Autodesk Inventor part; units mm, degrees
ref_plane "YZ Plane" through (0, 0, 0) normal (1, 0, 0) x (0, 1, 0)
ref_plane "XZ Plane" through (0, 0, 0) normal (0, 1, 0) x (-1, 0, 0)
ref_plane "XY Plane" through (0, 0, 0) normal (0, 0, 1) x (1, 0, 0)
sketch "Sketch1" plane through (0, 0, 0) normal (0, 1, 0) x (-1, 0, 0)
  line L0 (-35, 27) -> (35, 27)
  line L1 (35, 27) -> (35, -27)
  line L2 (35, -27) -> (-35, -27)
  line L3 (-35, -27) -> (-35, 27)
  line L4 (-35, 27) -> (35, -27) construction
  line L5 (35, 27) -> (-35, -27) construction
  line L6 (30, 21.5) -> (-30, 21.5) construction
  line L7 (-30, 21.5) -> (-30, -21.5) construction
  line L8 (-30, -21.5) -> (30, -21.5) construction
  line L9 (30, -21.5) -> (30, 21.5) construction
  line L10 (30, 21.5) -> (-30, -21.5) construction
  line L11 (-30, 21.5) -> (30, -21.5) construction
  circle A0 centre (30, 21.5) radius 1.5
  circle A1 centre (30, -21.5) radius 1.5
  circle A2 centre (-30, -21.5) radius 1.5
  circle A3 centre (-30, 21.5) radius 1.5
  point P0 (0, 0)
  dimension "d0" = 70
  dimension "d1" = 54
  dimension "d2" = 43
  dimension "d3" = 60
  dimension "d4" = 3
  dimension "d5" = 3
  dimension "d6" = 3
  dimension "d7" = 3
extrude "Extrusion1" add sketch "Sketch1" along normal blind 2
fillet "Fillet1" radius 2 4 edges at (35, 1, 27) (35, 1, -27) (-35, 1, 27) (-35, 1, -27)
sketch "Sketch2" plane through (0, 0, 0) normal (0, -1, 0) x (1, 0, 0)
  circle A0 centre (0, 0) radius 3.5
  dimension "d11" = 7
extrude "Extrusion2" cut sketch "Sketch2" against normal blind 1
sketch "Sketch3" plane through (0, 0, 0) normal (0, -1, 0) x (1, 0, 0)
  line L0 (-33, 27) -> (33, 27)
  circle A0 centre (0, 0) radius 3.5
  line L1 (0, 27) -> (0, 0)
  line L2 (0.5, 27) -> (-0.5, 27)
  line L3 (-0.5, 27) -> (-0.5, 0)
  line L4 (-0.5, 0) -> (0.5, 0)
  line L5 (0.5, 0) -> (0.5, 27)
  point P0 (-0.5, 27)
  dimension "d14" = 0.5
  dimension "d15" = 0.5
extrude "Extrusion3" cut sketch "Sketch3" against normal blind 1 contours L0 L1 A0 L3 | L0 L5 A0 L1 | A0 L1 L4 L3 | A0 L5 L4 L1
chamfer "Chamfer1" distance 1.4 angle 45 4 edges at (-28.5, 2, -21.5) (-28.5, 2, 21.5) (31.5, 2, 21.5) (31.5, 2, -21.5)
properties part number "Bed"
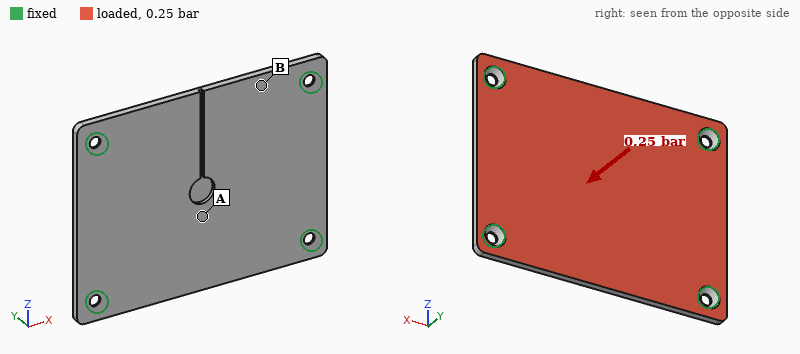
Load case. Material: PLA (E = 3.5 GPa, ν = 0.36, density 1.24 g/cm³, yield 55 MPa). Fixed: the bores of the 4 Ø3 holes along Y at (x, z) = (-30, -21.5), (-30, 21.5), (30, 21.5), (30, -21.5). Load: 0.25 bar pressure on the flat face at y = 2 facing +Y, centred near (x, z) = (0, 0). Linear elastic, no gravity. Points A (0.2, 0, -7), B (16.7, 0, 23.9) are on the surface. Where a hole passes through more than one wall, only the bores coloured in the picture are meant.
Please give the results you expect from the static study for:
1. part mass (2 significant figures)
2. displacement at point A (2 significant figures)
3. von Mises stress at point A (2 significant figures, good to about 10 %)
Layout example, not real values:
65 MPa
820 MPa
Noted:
9.2 g
0.78 mm
8.5 MPa
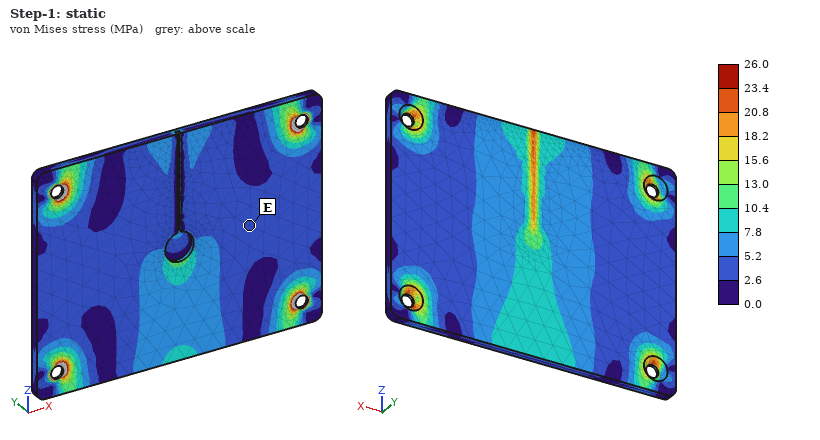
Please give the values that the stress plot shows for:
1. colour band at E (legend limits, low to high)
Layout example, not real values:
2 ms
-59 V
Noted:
2.6 to 5.2 MPa
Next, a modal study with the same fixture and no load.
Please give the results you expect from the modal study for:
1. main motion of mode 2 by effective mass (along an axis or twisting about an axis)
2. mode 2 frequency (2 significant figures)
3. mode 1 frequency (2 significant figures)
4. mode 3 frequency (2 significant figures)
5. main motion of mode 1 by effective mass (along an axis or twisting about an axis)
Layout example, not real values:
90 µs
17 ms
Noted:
twisting about X
1000 Hz
660 Hz
1500 Hz
along Y
